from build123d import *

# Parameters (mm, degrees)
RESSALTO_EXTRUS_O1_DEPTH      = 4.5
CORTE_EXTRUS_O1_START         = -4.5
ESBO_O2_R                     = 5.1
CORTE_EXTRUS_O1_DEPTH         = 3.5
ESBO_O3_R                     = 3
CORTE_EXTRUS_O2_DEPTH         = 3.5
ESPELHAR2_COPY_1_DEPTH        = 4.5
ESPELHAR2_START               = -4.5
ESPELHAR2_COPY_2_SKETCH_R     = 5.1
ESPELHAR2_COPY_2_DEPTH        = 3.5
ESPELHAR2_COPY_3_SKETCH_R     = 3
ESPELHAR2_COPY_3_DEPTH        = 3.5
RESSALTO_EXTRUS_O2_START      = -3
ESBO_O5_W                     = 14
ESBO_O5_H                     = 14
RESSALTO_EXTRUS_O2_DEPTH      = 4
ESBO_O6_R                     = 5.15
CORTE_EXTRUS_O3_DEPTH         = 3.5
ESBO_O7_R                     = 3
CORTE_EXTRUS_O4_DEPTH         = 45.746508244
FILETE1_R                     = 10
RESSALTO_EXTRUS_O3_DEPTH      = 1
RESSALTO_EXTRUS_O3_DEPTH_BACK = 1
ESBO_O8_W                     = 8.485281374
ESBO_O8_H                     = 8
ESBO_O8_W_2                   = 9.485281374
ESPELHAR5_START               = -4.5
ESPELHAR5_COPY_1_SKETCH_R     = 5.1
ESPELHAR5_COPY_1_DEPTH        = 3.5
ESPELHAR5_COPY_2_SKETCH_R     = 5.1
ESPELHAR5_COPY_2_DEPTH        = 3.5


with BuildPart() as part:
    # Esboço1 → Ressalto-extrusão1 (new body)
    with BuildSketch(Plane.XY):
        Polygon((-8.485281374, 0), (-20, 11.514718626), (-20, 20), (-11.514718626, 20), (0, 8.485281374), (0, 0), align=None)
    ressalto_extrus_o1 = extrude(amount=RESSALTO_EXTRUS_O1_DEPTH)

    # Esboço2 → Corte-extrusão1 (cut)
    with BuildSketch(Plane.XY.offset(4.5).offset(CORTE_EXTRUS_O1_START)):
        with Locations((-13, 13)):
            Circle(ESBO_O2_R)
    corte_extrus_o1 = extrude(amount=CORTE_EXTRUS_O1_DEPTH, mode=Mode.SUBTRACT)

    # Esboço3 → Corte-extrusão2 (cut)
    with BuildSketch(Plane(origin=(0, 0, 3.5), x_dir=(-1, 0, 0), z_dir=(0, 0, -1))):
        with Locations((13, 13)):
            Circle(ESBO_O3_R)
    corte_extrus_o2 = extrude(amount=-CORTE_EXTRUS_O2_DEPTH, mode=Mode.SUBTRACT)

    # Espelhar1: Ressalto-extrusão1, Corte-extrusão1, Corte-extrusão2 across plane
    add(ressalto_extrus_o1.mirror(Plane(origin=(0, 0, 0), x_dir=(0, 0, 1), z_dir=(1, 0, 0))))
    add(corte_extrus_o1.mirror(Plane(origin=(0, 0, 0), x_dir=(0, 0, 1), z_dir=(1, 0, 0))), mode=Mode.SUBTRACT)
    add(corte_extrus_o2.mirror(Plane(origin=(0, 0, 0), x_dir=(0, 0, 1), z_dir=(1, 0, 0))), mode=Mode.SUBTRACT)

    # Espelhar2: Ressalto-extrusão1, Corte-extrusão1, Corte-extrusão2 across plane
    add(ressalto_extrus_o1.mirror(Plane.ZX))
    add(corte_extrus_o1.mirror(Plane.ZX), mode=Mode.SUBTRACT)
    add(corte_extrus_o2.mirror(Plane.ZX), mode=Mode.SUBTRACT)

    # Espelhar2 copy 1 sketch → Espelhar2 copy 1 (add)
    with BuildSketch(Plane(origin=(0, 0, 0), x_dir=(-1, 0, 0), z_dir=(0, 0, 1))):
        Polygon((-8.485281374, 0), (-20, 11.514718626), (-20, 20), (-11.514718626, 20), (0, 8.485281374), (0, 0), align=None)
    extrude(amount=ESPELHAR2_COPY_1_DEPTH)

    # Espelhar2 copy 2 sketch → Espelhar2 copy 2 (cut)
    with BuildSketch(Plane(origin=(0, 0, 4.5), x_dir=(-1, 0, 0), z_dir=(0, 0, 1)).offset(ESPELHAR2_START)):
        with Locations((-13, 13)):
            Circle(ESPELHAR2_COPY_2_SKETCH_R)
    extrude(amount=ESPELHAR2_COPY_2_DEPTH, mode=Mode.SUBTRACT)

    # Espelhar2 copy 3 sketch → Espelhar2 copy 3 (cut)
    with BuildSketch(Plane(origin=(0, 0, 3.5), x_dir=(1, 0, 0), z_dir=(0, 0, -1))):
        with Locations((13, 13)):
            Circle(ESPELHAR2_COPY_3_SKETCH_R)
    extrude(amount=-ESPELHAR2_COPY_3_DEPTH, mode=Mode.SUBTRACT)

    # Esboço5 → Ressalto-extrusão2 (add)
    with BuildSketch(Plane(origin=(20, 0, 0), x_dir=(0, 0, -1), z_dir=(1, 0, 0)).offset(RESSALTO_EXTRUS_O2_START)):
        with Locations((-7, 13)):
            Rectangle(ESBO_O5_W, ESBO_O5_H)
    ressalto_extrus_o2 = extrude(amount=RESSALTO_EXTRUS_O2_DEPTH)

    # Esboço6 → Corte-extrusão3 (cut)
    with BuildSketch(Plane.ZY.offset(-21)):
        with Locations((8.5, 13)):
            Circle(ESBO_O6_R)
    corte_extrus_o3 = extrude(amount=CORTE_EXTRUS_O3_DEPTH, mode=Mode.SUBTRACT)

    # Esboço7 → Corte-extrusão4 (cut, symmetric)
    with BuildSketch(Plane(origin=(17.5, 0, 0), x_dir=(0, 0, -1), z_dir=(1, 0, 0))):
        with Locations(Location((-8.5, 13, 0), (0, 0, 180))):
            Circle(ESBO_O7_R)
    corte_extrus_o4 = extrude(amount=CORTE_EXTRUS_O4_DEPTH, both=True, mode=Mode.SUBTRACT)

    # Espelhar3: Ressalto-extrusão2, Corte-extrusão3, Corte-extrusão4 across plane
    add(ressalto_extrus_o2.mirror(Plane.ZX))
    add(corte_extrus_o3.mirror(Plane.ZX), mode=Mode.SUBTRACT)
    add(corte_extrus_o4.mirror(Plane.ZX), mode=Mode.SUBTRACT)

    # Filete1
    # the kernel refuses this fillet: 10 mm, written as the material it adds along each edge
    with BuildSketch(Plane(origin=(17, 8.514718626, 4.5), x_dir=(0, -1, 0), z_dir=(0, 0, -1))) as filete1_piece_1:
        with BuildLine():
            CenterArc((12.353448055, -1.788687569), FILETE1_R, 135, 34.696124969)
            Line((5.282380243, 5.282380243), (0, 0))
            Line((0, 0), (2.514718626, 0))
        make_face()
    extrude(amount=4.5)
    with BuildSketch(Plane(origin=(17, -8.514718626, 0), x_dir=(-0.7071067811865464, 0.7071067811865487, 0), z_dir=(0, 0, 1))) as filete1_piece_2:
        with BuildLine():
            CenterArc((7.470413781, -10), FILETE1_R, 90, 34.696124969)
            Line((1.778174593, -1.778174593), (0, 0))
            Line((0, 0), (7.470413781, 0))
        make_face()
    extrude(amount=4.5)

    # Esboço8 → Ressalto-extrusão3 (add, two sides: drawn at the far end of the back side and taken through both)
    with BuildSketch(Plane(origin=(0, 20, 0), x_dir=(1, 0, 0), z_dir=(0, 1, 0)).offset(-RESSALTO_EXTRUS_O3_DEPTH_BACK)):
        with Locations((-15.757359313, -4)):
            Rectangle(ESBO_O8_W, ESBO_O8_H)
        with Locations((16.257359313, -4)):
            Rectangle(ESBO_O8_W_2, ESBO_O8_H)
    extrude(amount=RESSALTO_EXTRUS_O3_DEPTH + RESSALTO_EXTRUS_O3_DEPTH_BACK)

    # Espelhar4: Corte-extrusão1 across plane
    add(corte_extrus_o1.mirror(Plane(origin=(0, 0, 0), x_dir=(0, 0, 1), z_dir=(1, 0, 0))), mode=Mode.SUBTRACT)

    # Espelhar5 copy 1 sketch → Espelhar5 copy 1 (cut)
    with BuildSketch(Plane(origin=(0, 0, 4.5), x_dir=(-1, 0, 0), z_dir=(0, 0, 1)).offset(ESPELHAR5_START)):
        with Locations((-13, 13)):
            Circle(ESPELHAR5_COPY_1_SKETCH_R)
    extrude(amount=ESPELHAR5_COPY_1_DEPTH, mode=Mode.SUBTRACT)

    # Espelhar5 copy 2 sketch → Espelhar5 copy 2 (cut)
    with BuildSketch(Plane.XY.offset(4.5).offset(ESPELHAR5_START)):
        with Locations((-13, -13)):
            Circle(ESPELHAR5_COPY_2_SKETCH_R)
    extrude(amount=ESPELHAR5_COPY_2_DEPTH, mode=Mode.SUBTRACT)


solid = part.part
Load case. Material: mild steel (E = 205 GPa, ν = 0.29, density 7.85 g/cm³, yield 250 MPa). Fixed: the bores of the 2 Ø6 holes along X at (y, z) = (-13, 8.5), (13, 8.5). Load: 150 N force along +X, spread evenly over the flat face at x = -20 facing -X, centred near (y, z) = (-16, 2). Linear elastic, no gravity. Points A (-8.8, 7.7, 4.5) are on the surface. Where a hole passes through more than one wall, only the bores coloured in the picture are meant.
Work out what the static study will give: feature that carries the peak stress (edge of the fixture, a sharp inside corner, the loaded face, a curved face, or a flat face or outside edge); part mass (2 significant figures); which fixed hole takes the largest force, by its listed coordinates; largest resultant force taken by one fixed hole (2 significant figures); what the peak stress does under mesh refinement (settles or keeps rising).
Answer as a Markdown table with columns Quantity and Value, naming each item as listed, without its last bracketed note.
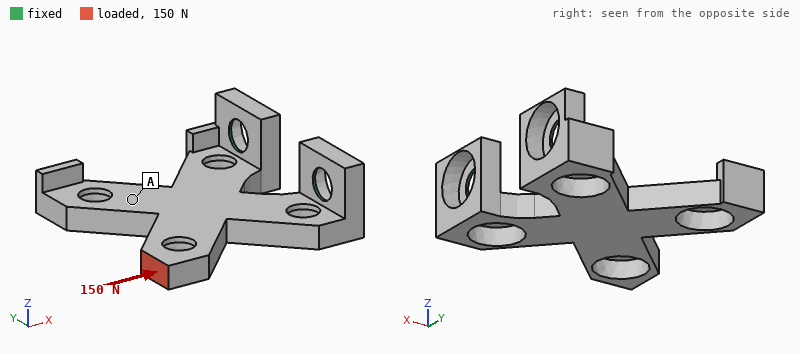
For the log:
| Quantity | Value |
|---|---|
| feature that carries the peak stress | edge of the fixture |
| part mass | 35 g |
| which fixed hole takes the largest force, by its listed coordinates | (-13, 8.5) |
| largest resultant force taken by one fixed hole | 160 N |
| what the peak stress does under mesh refinement | keeps rising |
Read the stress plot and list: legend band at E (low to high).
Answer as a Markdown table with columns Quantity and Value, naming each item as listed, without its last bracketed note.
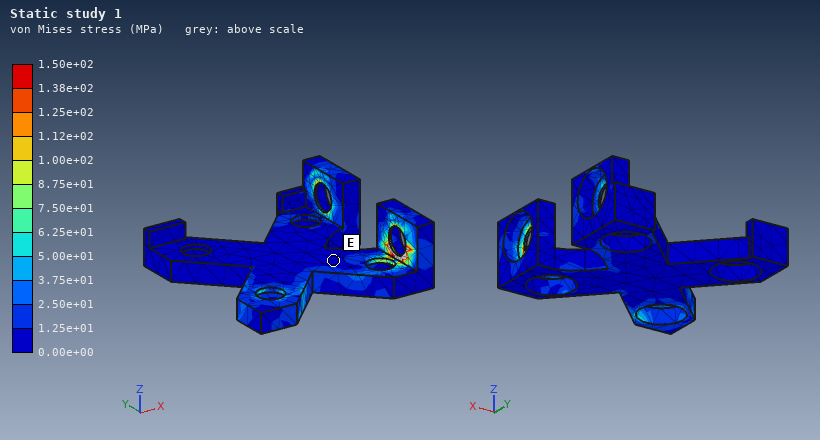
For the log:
| Quantity | Value |
|---|---|
| legend band at E | 0.00e+00 to 1.25e+01 MPa |
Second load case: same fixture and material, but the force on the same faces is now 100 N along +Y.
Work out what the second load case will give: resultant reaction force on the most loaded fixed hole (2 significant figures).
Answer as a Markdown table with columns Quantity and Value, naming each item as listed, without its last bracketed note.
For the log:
| Quantity | Value |
|---|---|
| resultant reaction force on the most loaded fixed hole | 140 N |
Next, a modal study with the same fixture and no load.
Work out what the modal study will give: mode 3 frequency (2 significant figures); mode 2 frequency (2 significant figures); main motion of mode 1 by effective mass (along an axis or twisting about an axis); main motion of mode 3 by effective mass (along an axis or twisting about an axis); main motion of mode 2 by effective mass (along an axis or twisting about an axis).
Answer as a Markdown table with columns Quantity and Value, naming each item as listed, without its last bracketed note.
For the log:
| Quantity | Value |
|---|---|
| mode 3 frequency | 4600 Hz |
| mode 2 frequency | 3300 Hz |
| main motion of mode 1 by effective mass | along Z |
| main motion of mode 3 by effective mass | along Y |
| main motion of mode 2 by effective mass | along Y |
